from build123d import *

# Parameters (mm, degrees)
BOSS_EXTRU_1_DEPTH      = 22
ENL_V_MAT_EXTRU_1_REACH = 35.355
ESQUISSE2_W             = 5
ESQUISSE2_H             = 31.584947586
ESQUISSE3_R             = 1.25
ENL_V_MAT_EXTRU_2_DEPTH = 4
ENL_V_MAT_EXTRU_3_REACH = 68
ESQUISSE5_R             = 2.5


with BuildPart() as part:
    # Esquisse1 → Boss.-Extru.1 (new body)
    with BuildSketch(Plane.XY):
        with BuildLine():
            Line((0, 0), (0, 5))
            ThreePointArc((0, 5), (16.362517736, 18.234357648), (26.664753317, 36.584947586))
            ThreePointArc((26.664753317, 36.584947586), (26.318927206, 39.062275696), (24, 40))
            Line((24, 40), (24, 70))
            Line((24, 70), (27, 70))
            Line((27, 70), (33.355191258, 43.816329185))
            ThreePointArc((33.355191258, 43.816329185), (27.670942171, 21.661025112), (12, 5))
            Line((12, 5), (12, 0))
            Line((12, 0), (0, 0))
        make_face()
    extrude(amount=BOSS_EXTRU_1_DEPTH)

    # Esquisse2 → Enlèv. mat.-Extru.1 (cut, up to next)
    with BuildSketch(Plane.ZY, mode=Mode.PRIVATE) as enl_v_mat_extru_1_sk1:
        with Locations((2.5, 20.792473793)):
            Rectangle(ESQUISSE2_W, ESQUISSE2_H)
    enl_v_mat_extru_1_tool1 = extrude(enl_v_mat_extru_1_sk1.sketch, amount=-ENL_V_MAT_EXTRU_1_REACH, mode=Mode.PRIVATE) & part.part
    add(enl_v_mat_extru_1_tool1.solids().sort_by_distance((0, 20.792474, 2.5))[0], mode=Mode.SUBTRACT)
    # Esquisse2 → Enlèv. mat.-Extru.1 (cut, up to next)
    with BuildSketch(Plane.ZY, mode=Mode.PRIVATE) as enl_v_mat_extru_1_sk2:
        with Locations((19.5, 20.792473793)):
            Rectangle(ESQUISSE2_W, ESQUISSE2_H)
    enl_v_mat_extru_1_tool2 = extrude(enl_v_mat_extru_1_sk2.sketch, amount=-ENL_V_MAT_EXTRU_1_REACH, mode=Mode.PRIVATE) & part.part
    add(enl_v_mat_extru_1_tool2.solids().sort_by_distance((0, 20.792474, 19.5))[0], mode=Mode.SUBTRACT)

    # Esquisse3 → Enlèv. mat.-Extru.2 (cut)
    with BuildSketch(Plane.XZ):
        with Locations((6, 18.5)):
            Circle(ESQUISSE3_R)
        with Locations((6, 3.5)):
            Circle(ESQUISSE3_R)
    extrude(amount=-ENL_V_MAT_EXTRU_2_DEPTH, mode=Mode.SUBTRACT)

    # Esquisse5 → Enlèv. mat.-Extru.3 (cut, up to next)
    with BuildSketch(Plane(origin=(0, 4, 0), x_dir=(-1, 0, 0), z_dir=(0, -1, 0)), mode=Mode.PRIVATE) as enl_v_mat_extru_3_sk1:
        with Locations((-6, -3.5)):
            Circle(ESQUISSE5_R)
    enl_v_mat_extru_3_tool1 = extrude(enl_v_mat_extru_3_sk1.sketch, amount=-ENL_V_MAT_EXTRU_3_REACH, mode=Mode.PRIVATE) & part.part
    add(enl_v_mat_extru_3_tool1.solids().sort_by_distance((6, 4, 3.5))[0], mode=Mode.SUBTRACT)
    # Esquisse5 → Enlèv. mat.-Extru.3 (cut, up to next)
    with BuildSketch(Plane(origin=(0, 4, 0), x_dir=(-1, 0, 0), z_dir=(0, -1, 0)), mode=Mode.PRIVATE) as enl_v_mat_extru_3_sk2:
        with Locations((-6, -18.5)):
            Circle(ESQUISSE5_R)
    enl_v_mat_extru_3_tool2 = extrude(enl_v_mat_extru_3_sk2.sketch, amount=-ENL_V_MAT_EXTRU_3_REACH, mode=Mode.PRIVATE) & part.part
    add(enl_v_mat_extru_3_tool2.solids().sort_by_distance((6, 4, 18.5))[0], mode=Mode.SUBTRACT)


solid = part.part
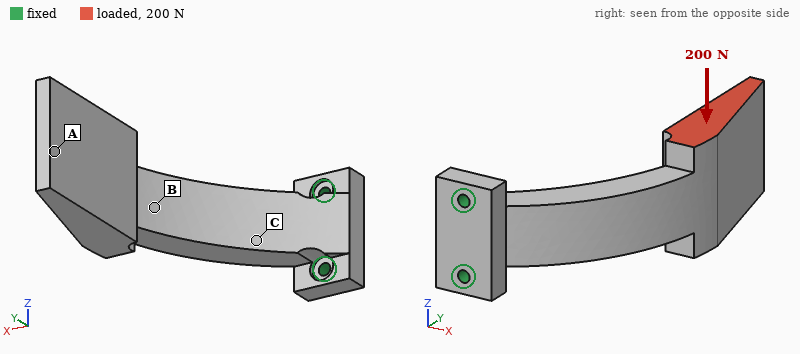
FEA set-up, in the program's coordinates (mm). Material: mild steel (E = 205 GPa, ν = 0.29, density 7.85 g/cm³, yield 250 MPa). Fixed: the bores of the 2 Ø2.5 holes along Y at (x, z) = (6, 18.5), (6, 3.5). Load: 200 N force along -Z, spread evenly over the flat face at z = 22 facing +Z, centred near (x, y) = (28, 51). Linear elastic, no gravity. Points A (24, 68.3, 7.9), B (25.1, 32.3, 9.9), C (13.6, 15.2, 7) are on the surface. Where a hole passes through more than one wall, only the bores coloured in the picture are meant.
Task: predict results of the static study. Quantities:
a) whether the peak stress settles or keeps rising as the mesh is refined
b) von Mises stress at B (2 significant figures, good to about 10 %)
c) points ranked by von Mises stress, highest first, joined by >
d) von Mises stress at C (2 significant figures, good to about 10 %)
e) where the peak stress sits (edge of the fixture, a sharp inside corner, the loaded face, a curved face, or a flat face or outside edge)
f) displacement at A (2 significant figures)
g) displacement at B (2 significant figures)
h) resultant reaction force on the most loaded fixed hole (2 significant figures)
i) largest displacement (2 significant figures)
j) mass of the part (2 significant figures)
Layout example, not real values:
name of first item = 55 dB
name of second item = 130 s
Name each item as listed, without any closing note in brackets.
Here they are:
whether the peak stress settles or keeps rising as the mesh is refined = keeps rising
von Mises stress at B = 27 MPa
points ranked by von Mises stress, highest first, joined by > = C > B > A
von Mises stress at C = 46 MPa
where the peak stress sits = edge of the fixture
displacement at A = 0.11 mm
displacement at B = 0.034 mm
resultant reaction force on the most loaded fixed hole = 770 N
largest displacement = 0.11 mm
mass of the part = 74 g
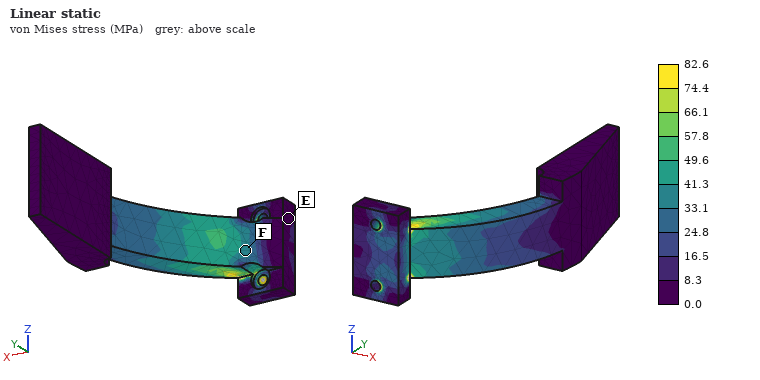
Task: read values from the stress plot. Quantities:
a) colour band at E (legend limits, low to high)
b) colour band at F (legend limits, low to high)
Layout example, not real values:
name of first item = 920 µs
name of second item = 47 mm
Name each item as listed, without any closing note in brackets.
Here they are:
colour band at E = 0.0 to 8.3 MPa
colour band at F = 33.1 to 41.3 MPa
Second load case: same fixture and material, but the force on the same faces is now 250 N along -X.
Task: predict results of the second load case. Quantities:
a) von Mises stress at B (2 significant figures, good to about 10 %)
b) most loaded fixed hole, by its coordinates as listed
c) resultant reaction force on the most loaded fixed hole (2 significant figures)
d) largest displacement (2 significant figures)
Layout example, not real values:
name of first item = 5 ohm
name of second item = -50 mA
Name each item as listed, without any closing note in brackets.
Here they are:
von Mises stress at B = 66 MPa
most loaded fixed hole, by its coordinates as listed = (6, 18.5)
resultant reaction force on the most loaded fixed hole = 320 N
largest displacement = 0.35 mm
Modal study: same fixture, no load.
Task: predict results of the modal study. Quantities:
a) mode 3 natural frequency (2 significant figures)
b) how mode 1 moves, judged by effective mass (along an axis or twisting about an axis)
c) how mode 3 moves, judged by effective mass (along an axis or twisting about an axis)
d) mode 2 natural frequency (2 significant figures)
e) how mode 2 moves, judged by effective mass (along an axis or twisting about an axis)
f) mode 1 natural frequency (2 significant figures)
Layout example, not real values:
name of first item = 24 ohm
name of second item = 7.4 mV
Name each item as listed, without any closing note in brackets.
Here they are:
mode 3 natural frequency = 3900 Hz
how mode 1 moves, judged by effective mass = along X
how mode 3 moves, judged by effective mass = along Y
mode 2 natural frequency = 1300 Hz
how mode 2 moves, judged by effective mass = along Z
mode 1 natural frequency = 790 Hz
